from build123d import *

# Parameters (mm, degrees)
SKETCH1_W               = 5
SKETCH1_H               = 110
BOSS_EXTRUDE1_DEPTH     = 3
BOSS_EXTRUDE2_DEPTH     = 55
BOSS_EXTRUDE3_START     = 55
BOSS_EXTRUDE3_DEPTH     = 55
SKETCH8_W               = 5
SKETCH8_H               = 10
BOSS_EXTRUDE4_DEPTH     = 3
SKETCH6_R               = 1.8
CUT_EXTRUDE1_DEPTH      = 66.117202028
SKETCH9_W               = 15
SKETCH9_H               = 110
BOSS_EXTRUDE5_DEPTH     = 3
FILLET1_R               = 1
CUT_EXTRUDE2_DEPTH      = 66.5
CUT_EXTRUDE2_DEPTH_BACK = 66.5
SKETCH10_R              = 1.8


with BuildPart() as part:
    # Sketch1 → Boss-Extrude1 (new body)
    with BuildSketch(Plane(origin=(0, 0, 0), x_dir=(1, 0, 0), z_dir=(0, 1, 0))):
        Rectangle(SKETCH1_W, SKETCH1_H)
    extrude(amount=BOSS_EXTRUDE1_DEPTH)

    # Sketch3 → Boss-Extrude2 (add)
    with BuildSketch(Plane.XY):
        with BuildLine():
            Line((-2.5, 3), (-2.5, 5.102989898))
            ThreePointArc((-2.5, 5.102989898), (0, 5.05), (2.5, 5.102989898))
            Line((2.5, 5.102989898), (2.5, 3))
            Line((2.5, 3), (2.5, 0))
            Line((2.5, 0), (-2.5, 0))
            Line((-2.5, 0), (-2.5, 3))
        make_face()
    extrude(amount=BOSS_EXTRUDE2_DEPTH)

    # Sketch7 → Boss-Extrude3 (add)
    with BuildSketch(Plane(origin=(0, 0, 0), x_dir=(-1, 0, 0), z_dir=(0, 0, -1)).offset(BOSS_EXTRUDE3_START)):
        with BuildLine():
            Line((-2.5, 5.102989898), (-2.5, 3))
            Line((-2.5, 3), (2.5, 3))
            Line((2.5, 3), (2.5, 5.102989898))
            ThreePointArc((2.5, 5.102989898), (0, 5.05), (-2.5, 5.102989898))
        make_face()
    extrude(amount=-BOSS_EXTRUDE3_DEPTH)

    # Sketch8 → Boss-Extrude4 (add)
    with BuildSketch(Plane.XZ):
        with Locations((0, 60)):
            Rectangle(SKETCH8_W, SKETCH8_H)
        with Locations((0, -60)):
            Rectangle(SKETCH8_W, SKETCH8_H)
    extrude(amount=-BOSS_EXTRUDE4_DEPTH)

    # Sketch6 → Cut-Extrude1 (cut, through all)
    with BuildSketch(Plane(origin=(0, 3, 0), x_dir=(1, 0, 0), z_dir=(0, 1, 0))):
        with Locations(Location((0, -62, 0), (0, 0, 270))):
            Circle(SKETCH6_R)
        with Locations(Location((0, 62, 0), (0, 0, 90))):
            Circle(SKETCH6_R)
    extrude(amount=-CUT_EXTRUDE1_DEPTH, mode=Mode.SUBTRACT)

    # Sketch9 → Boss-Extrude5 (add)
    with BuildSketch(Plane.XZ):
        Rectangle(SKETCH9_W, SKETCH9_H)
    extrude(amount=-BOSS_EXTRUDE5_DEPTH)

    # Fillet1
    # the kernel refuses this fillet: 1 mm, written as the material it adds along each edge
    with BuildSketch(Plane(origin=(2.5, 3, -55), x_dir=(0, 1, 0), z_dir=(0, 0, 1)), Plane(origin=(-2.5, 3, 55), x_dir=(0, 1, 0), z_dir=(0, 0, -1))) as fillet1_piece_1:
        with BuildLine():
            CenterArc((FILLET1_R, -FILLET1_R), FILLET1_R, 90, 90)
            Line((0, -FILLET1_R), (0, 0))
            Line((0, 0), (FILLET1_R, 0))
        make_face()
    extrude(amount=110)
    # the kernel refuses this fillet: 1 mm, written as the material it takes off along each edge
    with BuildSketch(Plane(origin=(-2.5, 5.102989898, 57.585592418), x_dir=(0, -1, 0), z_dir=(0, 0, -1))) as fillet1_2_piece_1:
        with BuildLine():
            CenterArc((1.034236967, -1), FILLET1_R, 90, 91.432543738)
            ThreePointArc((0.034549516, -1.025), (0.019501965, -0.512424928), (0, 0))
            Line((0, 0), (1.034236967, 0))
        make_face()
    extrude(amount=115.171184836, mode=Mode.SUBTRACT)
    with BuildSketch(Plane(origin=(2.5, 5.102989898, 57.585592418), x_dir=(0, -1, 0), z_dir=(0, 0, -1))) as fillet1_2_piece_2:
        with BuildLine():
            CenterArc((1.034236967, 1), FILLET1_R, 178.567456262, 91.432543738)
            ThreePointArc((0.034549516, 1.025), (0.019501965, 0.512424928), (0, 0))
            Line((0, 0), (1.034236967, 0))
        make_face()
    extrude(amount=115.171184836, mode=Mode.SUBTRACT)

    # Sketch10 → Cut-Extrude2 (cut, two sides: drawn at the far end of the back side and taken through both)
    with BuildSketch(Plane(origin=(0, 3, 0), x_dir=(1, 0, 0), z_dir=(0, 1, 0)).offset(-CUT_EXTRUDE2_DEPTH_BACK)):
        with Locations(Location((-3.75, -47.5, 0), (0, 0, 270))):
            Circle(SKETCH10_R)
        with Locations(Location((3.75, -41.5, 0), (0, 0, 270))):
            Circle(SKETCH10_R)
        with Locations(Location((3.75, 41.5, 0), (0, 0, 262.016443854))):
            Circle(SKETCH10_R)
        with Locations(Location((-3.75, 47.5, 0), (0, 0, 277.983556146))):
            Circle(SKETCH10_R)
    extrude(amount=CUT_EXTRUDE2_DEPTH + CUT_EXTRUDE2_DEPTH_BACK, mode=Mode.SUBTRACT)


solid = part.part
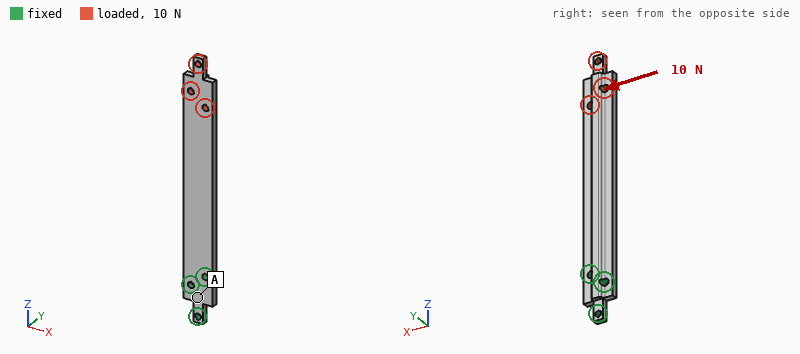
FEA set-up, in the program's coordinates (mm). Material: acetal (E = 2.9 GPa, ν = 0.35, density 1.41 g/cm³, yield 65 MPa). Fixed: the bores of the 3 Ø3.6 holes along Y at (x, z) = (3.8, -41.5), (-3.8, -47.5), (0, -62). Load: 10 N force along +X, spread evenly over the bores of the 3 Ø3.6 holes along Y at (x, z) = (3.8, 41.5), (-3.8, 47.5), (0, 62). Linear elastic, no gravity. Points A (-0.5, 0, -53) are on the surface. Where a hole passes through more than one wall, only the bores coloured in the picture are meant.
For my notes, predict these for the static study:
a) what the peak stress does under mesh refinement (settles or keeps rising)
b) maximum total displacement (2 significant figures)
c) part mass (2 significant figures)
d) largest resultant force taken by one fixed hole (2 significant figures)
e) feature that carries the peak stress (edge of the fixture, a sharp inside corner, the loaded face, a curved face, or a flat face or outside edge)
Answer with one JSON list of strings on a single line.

["keeps rising", "1.4 mm", "8.7 g", "87 N", "edge of the fixture"]
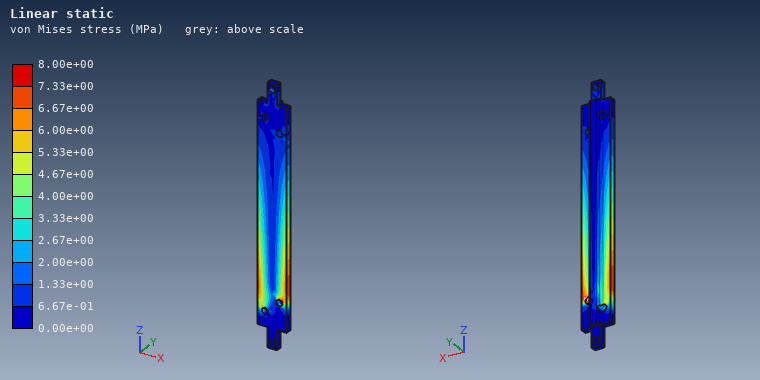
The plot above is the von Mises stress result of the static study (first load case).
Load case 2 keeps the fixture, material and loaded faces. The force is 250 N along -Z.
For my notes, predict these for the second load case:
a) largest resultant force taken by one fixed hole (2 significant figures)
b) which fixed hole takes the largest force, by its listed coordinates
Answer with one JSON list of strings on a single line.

["140 N", "(3.8, -41.5)"]
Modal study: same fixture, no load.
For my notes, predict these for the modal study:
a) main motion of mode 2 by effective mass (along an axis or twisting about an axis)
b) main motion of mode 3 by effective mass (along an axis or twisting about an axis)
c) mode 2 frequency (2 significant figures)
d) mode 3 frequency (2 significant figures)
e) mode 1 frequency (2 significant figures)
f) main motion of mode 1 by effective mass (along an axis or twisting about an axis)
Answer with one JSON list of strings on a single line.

["along X", "along Y", "310 Hz", "630 Hz", "100 Hz", "along Y"]
